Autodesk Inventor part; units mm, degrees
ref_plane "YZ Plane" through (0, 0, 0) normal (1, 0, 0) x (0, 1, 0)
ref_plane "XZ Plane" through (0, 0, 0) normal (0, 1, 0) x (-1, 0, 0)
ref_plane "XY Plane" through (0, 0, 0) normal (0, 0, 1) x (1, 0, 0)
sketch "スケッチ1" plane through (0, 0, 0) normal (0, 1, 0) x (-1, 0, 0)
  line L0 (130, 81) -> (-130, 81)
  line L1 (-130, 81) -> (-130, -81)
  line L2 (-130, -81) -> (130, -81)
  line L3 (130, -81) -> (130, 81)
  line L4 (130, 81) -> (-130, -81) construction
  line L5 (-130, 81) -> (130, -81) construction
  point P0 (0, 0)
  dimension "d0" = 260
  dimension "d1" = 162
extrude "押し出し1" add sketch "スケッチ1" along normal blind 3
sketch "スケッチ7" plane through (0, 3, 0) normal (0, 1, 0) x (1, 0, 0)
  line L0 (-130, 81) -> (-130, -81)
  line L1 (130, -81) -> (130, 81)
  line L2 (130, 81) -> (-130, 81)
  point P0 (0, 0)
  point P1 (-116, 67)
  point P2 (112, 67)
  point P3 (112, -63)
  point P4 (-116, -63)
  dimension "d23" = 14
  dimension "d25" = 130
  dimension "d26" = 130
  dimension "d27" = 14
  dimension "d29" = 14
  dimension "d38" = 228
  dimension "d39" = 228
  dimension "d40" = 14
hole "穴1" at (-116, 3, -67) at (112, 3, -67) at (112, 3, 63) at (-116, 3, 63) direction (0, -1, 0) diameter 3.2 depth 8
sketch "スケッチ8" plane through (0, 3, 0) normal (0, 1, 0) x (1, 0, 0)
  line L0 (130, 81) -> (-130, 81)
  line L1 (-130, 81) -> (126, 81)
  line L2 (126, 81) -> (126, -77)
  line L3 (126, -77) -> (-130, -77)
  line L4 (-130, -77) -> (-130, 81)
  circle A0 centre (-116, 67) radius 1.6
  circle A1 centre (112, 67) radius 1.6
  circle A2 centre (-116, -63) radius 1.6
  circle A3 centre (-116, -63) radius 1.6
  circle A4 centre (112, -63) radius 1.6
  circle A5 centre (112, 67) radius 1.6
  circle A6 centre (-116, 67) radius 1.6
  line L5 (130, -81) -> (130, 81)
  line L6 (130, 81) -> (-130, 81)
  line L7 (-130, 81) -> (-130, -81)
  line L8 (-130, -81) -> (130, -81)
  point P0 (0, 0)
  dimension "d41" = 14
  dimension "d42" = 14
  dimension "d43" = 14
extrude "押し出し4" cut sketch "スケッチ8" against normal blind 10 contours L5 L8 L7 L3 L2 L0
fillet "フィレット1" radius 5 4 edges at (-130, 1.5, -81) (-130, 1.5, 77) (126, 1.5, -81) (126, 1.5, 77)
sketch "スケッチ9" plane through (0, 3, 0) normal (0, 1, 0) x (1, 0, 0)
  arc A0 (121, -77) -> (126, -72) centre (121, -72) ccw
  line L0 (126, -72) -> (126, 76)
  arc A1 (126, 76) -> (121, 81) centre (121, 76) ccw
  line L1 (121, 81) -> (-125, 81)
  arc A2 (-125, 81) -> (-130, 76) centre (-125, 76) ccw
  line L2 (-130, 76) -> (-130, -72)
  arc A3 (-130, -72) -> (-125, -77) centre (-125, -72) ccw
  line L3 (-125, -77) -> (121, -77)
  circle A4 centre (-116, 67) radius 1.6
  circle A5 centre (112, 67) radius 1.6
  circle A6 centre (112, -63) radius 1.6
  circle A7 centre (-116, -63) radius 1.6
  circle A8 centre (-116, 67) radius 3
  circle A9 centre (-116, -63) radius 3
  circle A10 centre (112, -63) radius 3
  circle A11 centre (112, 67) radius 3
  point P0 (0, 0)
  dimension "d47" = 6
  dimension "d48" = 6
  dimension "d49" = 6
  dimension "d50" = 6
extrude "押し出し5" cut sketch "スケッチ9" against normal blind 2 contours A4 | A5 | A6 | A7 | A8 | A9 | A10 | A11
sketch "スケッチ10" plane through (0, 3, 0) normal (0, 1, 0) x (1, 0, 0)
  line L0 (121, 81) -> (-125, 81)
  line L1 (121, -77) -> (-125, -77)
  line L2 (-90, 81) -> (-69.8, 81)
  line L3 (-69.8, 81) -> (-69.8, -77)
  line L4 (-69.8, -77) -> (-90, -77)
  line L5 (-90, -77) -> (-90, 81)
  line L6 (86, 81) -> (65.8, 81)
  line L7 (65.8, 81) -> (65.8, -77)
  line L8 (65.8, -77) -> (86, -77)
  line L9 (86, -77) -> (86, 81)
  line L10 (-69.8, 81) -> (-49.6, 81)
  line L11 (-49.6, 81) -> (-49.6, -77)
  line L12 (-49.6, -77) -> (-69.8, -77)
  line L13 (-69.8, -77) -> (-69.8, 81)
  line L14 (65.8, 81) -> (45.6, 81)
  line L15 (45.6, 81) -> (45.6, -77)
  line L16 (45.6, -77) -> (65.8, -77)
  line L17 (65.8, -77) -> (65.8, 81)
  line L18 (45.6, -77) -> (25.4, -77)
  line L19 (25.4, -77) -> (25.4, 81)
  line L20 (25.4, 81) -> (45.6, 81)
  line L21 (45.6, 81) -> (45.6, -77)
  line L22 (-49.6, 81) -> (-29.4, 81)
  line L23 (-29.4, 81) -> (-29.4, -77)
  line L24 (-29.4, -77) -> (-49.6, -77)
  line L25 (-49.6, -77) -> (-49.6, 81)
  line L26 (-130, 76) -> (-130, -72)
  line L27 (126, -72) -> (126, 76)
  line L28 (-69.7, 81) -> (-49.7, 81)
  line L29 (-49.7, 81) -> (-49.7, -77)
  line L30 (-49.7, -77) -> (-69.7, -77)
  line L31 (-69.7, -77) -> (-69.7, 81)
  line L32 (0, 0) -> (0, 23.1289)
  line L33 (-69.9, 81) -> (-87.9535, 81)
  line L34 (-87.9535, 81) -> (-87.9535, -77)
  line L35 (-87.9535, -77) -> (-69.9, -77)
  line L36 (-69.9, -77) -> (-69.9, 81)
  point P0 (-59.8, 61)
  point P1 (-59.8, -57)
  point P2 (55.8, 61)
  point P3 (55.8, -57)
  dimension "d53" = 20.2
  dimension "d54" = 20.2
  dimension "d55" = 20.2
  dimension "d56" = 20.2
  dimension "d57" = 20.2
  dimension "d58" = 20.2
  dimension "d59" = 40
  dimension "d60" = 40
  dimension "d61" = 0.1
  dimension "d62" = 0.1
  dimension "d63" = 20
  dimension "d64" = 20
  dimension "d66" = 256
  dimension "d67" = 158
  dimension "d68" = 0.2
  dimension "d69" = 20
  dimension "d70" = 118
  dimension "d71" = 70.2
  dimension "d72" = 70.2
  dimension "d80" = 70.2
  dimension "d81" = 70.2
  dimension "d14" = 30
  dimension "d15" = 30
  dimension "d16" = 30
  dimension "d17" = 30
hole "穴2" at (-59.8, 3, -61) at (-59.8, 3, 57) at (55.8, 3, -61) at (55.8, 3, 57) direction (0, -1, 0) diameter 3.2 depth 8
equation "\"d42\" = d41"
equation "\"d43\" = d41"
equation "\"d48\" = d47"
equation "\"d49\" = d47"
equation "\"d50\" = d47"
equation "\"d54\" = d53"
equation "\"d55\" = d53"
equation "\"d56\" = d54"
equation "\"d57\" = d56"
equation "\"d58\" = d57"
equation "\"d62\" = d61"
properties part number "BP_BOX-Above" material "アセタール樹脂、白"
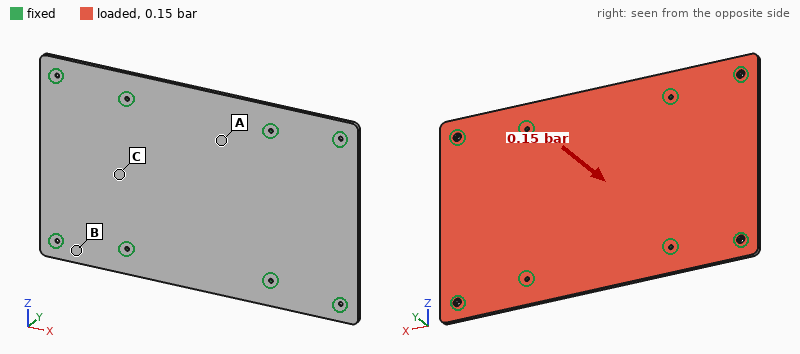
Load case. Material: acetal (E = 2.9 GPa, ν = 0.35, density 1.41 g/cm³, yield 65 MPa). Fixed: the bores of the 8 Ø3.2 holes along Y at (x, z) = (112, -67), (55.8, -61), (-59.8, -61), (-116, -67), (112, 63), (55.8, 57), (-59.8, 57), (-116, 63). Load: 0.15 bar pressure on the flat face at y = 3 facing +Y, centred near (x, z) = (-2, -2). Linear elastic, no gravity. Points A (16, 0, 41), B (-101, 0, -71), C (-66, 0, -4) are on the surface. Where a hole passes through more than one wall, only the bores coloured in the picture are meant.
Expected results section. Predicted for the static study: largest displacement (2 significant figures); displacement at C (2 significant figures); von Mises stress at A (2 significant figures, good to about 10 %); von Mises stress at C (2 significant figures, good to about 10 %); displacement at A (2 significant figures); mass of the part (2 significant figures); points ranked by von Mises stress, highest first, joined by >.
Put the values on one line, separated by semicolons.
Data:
2.9 mm; 2.1 mm; 4.8 MPa; 8.3 MPa; 1.8 mm; 170 g; C > A > B
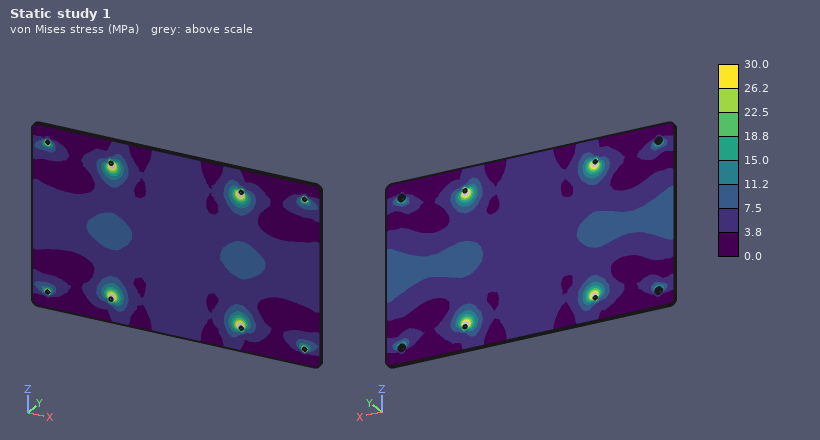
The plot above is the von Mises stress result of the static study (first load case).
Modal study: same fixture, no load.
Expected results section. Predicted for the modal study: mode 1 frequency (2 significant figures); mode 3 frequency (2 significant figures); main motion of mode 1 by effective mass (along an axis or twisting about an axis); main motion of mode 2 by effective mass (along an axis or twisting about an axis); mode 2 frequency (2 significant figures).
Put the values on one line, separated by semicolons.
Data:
210 Hz; 240 Hz; along Y; twisting about Z; 230 Hz
